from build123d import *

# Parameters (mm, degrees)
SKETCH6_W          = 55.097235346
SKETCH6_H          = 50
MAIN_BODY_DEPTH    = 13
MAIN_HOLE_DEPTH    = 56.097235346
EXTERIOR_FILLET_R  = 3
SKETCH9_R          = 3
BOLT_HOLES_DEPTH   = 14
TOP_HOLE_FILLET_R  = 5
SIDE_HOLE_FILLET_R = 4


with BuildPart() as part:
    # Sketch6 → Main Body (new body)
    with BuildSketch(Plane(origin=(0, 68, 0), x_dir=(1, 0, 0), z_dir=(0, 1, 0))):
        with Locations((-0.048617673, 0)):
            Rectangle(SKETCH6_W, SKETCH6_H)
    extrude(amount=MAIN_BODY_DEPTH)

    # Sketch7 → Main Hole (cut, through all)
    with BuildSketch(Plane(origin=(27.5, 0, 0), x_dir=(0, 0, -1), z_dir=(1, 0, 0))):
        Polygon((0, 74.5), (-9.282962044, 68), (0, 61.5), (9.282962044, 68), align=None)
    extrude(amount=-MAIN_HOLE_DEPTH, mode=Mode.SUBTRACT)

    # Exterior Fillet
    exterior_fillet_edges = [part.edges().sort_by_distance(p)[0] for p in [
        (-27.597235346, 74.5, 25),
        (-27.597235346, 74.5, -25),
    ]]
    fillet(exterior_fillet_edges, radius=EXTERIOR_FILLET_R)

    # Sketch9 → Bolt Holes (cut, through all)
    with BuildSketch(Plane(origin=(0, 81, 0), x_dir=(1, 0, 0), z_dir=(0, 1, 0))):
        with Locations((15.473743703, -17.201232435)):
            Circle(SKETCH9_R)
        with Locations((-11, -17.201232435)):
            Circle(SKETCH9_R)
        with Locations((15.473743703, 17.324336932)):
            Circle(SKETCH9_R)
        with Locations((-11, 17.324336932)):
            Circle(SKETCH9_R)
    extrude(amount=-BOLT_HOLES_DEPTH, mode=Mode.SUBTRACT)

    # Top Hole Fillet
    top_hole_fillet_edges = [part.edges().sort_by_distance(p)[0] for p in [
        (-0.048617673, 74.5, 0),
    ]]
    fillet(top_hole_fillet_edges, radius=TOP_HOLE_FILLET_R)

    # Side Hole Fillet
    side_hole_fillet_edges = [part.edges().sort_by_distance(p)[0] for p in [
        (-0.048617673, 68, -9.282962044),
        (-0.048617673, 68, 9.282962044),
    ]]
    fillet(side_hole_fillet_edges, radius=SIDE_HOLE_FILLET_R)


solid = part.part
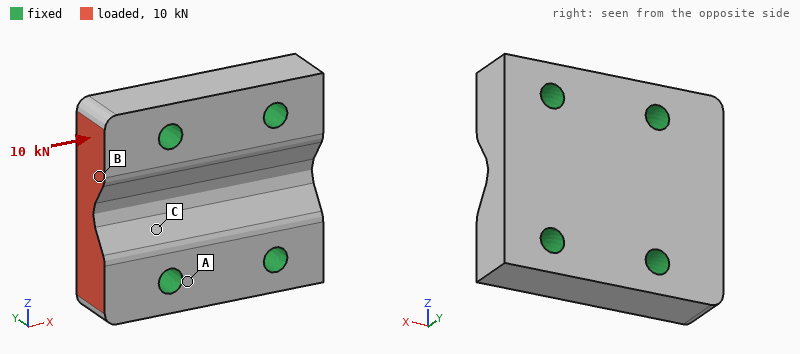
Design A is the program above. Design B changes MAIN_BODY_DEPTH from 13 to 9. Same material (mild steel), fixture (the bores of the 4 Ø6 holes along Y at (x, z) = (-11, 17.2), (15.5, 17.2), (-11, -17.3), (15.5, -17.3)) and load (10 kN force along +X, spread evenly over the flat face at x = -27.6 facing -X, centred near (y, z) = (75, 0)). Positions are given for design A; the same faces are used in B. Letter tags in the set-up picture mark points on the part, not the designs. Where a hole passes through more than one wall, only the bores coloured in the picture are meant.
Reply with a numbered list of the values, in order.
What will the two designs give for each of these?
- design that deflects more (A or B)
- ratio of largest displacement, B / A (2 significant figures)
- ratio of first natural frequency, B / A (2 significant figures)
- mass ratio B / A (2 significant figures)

1. B
2. 1.7
3. 0.84
4. 0.66
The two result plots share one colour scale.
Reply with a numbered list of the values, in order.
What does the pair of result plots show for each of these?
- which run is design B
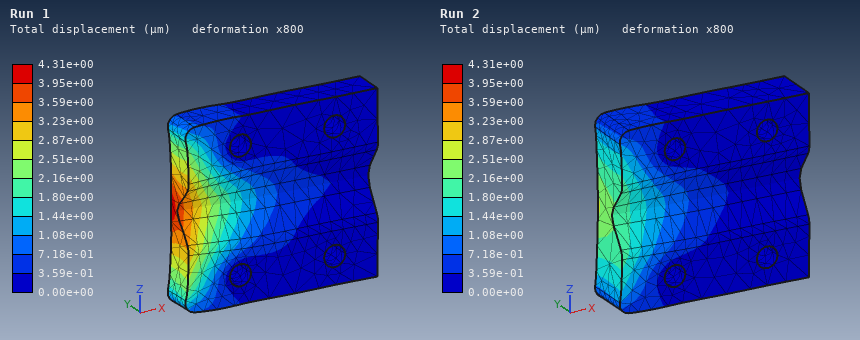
1. Run 1
